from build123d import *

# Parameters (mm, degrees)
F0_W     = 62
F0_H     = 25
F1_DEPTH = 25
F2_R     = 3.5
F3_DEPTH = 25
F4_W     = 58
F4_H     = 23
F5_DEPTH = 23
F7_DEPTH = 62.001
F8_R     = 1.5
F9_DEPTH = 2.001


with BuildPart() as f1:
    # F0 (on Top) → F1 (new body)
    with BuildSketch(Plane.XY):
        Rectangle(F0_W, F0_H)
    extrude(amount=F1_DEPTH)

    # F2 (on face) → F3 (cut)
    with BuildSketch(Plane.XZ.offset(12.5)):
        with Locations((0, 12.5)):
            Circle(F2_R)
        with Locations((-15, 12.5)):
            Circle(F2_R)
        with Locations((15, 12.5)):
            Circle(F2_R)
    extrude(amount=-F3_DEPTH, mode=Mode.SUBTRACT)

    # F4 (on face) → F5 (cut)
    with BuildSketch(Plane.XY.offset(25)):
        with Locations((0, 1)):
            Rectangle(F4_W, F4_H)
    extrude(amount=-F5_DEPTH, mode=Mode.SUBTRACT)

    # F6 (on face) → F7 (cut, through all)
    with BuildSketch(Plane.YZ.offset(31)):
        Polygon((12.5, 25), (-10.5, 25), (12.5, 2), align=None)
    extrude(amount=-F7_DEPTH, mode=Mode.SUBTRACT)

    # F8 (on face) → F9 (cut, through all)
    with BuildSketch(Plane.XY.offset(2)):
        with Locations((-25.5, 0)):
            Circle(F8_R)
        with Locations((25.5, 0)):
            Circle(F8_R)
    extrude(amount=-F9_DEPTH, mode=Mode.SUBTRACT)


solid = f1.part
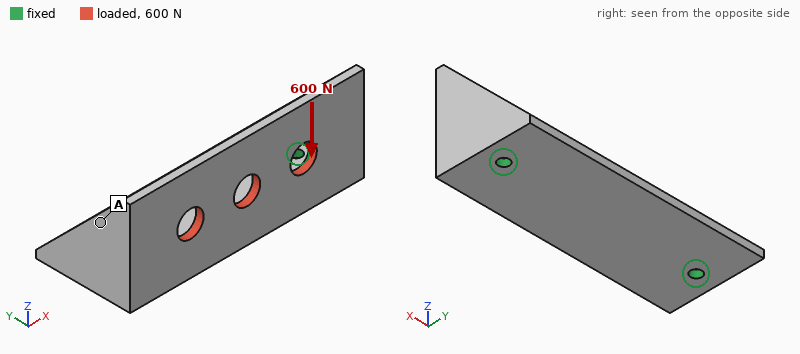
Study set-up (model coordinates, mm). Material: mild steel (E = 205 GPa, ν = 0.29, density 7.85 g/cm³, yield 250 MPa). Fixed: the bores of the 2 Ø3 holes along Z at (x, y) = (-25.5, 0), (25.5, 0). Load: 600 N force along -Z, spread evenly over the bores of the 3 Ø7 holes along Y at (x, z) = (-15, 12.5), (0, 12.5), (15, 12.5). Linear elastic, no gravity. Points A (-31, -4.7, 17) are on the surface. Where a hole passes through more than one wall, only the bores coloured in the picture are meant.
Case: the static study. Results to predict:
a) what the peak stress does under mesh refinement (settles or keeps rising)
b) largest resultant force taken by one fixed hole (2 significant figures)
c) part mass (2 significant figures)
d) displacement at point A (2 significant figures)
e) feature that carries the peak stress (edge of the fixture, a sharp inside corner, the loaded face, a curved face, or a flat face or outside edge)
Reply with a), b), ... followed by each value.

a) keeps rising
b) 300 N
c) 53 g
d) 42 µm
e) edge of the fixture
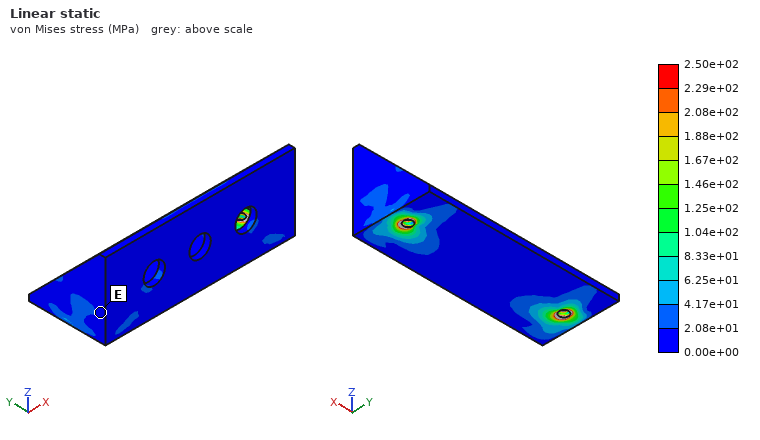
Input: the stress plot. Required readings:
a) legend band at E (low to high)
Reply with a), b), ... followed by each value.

a) 0.00e+00 to 2.08e+01 MPa
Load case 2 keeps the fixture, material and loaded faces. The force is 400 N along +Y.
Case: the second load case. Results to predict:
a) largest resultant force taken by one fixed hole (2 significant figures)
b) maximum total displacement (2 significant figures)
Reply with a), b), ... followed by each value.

a) 210 N
b) 0.12 mm
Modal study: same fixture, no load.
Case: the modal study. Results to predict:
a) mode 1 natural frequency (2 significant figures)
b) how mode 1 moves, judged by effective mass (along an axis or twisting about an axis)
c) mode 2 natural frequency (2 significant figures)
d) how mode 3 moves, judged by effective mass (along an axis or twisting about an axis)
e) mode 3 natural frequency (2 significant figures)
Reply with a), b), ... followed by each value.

a) 2400 Hz
b) along Y
c) 3600 Hz
d) along Z
e) 4500 Hz
